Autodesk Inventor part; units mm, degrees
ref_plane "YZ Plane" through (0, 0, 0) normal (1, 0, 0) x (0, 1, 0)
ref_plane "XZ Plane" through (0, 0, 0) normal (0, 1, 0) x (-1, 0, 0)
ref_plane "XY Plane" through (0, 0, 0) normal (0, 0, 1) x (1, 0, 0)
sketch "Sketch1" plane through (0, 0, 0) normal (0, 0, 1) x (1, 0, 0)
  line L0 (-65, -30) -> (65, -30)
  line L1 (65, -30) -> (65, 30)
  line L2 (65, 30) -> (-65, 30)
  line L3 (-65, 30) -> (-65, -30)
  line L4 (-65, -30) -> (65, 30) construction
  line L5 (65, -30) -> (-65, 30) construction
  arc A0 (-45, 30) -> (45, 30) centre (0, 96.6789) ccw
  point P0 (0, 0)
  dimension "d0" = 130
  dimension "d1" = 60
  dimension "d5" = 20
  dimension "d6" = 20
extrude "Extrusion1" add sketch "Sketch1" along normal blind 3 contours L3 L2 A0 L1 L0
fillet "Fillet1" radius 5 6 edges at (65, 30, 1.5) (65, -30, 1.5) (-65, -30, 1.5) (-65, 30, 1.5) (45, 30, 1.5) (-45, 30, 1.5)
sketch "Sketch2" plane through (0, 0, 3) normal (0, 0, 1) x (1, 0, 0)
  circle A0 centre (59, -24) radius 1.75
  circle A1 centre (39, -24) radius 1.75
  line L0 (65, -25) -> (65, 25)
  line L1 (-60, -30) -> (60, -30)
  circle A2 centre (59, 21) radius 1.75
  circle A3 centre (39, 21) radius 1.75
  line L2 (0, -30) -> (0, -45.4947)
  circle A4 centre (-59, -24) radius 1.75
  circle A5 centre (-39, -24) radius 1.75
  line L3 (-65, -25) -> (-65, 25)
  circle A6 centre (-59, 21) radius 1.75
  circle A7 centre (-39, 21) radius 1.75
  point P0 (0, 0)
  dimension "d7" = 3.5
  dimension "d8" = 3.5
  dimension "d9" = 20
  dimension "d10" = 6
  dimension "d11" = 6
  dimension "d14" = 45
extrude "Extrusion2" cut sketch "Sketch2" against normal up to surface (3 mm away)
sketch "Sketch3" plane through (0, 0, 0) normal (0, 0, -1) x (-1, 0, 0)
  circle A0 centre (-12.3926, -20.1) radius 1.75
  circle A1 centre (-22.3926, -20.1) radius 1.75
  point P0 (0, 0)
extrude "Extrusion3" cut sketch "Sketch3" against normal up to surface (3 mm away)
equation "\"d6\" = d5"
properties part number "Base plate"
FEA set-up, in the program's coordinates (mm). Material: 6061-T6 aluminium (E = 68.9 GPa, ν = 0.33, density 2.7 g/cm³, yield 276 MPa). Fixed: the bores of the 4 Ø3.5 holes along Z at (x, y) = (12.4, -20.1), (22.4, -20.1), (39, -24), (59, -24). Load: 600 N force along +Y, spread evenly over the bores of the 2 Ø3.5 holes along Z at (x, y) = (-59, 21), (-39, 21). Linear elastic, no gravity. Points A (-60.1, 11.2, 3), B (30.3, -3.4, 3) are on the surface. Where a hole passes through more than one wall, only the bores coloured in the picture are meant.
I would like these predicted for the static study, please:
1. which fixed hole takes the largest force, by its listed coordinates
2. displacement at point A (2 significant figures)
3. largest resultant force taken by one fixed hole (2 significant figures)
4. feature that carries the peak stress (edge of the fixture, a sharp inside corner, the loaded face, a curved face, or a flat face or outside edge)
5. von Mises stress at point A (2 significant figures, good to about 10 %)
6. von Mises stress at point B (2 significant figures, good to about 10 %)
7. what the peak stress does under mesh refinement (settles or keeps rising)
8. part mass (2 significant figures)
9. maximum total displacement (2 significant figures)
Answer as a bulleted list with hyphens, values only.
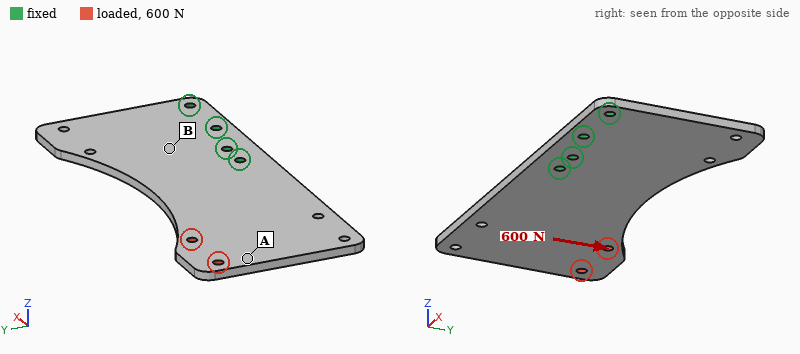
- (12.4, -20.1)
- 0.095 mm
- 1.5 kN
- edge of the fixture
- 6.7 MPa
- 16 MPa
- keeps rising
- 55 g
- 0.11 mm
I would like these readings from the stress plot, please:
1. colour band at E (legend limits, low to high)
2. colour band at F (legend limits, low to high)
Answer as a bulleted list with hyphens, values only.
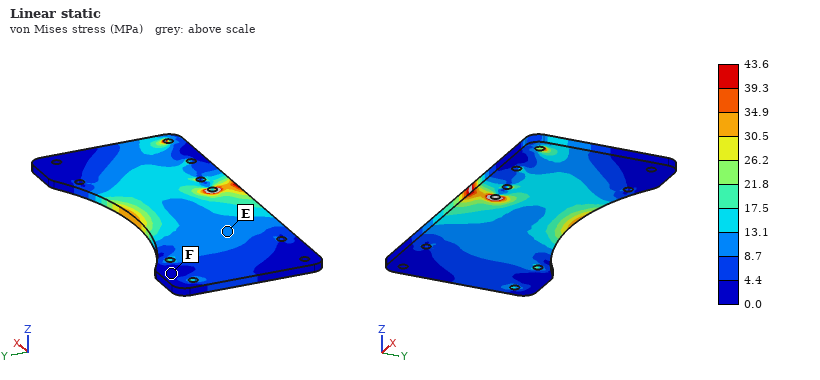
- 8.7 to 13.1 MPa
- 0.0 to 4.4 MPa
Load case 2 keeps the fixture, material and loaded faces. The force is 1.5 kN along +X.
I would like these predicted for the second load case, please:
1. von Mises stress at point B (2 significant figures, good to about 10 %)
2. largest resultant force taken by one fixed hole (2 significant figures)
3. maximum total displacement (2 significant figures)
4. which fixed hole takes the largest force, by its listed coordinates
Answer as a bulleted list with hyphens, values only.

- 28 MPa
- 1.5 kN
- 0.17 mm
- (12.4, -20.1)
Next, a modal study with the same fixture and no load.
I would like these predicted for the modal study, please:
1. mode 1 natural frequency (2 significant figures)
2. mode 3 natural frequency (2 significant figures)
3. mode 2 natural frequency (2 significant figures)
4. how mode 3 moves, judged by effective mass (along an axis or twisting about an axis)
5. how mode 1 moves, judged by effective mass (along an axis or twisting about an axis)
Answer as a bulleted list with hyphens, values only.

- 330 Hz
- 1200 Hz
- 900 Hz
- along Z
- along Z
